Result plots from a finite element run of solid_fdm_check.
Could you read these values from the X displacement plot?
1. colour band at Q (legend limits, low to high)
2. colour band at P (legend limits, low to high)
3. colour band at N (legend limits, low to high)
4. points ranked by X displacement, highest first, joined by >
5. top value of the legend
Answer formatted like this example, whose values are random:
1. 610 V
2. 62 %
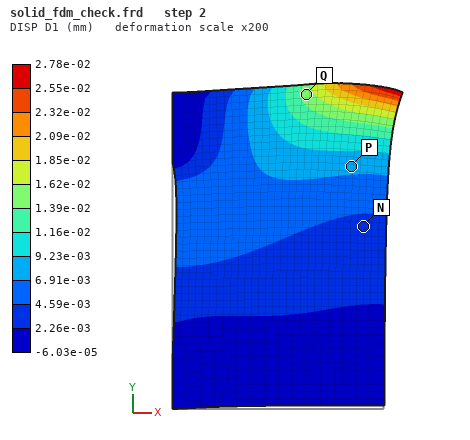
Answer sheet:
1. 1.39e-02 to 1.62e-02 mm
2. 6.91e-03 to 9.23e-03 mm
3. 2.26e-03 to 4.59e-03 mm
4. Q > P > N
5. 2.78e-02 mm
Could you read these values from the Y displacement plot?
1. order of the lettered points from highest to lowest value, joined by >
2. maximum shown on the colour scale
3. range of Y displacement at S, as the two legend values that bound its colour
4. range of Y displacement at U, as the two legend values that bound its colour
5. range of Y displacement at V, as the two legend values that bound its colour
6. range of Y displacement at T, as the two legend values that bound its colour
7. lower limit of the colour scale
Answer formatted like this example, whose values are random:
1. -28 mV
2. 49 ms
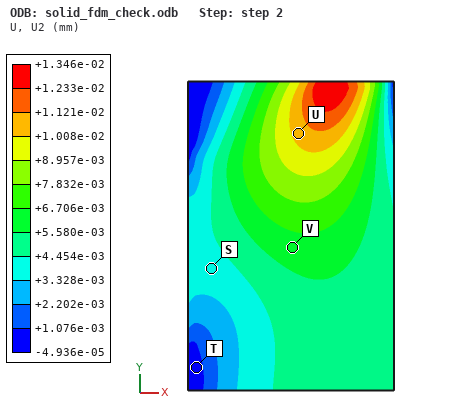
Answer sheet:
1. U > V > S > T
2. +1.346e-02 mm
3. +3.328e-03 to +4.454e-03 mm
4. +1.008e-02 to +1.121e-02 mm
5. +5.580e-03 to +6.706e-03 mm
6. -4.936e-05 to +1.076e-03 mm
7. -4.936e-05 mm
